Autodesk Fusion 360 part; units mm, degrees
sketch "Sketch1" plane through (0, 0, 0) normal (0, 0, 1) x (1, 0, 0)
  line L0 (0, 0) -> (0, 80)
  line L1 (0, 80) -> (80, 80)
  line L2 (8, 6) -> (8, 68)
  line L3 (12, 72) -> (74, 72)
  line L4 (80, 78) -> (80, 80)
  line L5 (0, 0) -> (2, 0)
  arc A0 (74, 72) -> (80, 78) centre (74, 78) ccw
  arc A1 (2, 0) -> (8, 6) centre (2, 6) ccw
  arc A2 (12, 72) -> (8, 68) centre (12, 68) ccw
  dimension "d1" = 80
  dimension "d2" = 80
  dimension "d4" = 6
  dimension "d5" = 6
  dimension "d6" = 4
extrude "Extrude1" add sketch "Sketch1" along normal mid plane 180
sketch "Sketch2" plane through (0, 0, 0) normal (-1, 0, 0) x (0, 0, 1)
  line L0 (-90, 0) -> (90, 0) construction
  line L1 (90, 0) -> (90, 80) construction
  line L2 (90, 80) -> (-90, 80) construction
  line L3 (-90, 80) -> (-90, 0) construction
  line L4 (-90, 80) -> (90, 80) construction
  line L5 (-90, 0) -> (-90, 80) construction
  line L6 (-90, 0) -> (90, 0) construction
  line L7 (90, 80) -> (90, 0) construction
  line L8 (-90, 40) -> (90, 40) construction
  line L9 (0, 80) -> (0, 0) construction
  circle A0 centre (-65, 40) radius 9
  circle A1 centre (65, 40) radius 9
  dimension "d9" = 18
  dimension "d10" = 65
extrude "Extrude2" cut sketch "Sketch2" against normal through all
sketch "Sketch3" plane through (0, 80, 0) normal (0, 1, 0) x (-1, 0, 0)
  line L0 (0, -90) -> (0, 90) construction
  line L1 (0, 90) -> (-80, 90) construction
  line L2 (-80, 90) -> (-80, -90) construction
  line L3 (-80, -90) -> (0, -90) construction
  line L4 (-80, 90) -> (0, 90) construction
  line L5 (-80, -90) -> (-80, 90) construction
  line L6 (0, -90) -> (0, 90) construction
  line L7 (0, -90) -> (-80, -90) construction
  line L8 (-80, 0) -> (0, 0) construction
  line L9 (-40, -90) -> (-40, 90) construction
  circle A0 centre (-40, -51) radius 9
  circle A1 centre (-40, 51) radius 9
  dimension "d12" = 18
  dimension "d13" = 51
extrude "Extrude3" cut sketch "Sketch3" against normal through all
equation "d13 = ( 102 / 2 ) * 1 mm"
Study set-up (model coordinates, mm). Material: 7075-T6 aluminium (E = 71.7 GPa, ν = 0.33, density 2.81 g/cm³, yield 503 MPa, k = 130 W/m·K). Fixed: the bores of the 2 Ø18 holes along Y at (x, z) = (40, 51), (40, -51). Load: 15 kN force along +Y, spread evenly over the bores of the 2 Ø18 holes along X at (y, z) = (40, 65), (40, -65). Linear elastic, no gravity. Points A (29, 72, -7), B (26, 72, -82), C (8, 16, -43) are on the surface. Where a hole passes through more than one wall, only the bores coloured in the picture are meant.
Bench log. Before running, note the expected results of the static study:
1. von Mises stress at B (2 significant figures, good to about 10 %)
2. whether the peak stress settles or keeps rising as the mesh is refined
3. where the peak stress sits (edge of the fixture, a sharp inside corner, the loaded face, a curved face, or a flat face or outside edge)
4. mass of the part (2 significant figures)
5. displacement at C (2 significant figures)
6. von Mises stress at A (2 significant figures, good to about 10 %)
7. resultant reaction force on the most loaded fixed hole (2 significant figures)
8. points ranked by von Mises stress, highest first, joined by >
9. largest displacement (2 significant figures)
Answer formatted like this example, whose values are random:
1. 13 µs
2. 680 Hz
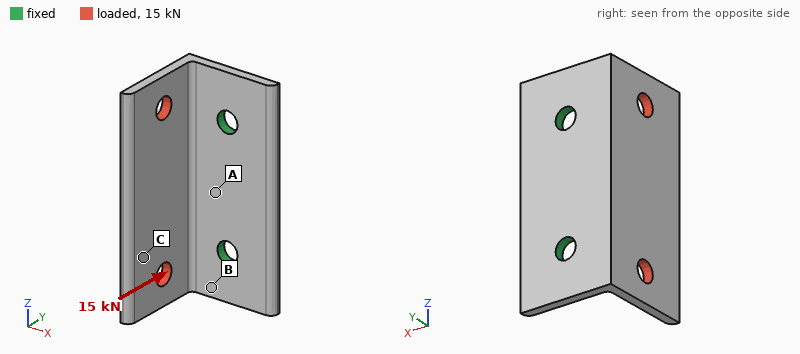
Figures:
1. 110 MPa
2. keeps rising
3. edge of the fixture
4. 590 g
5. 0.93 mm
6. 76 MPa
7. 7.5 kN
8. B > A > C
9. 1.2 mm
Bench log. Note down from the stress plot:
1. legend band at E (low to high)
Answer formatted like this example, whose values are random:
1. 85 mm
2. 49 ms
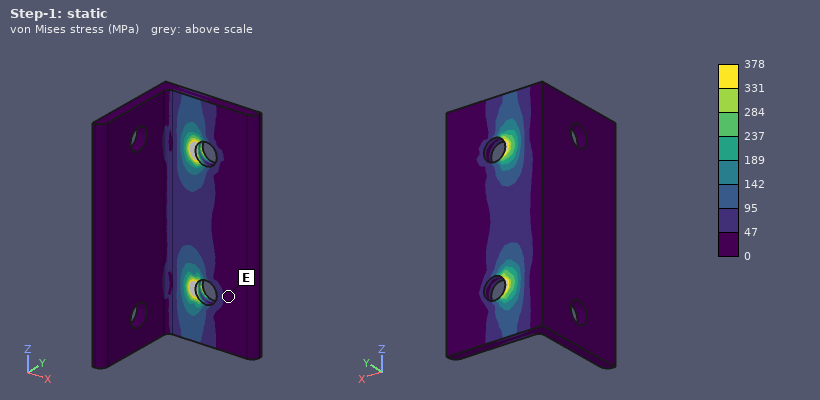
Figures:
1. 0 to 47 MPa
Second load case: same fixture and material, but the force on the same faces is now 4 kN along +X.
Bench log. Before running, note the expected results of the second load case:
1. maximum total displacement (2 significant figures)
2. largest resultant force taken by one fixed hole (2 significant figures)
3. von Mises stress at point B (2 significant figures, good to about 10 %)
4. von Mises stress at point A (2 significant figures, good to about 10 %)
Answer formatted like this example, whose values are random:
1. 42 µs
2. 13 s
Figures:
1. 0.90 mm
2. 2.0 kN
3. 65 MPa
4. 40 MPa
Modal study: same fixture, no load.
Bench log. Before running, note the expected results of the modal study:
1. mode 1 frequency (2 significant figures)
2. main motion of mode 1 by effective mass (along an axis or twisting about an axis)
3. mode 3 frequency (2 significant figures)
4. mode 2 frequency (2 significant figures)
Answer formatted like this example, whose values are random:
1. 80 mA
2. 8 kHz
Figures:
1. 720 Hz
2. along X
3. 2200 Hz
4. 1200 Hz
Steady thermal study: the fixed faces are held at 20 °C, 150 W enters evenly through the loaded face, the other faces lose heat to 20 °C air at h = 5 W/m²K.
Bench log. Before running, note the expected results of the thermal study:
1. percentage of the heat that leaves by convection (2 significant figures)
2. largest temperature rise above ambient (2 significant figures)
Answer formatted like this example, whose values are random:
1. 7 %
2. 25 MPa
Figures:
1. 5.8 %
2. 74 K
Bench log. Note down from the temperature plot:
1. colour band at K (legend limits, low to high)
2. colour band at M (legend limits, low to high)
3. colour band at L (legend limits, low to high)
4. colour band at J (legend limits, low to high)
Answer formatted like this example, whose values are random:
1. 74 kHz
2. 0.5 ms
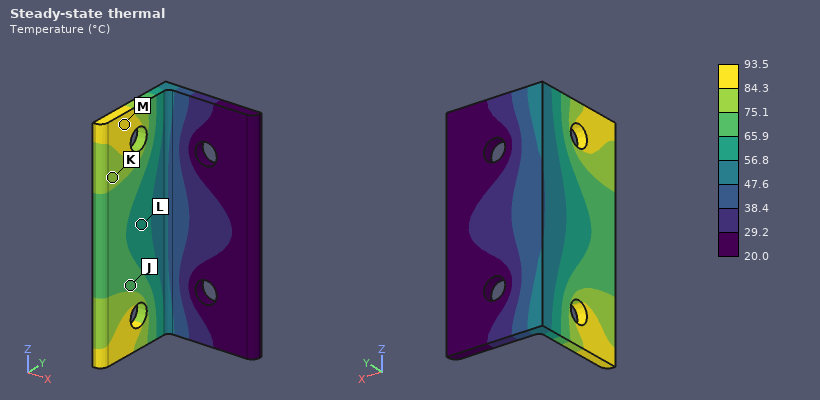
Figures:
1. 75.1 to 84.3 °C
2. 84.3 to 93.5 °C
3. 56.8 to 65.9 °C
4. 65.9 to 75.1 °C
